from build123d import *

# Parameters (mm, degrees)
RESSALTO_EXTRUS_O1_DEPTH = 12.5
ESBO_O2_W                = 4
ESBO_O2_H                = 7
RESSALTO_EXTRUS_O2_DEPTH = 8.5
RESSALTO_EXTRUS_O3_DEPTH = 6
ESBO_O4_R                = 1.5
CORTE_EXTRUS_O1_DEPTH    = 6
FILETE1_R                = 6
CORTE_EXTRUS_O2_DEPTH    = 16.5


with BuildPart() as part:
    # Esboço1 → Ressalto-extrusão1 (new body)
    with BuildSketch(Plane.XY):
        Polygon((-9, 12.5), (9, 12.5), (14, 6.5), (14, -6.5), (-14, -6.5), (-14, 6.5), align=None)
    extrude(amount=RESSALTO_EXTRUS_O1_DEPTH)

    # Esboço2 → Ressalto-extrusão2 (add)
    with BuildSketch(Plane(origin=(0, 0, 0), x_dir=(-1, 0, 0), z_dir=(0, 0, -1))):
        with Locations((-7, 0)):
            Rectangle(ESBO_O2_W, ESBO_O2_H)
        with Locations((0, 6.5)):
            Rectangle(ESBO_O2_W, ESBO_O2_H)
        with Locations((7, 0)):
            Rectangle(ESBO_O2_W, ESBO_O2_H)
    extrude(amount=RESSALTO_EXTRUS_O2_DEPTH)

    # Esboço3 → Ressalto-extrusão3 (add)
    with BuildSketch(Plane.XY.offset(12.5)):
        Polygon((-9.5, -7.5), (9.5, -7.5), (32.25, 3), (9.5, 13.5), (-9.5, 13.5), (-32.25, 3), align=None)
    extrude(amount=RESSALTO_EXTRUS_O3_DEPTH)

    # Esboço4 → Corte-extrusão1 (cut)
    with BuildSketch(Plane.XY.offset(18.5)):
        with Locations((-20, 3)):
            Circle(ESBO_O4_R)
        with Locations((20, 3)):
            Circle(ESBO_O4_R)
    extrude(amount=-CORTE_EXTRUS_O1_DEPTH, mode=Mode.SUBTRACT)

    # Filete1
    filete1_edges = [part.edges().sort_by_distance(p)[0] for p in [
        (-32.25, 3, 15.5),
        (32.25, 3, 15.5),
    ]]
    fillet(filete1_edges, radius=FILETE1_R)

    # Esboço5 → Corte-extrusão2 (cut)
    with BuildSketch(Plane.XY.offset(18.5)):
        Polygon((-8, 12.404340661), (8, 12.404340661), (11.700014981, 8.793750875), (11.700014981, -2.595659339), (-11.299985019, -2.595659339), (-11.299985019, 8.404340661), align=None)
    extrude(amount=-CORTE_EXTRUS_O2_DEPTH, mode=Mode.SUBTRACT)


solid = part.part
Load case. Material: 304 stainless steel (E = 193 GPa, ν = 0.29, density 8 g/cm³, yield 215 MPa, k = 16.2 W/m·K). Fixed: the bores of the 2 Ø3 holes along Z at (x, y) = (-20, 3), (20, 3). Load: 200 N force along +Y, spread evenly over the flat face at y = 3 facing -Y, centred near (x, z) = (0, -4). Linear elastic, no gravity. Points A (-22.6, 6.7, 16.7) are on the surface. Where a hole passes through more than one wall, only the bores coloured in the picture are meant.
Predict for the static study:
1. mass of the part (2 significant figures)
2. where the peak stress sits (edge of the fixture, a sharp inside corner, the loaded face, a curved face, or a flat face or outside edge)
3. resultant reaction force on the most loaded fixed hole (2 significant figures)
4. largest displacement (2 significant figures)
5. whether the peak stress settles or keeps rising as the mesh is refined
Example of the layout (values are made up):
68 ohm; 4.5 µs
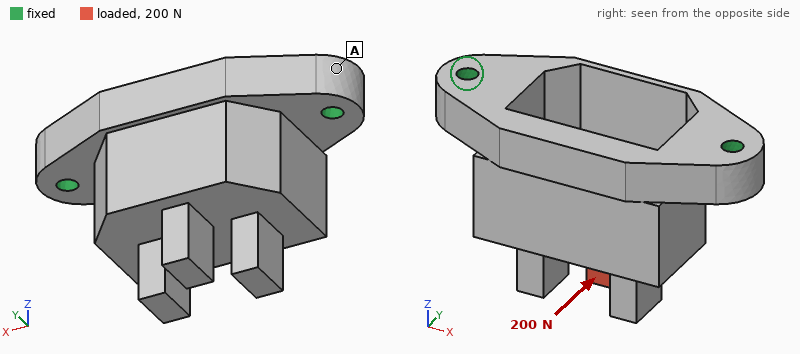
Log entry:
50 g; edge of the fixture; 110 N; 14 µm; keeps rising
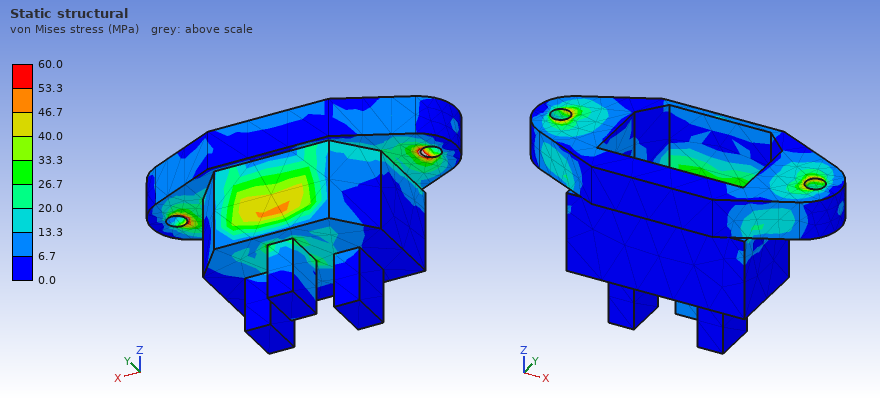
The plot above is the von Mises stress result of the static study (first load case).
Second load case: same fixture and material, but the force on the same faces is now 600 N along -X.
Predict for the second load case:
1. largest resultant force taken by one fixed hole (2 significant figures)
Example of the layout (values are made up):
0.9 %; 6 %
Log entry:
480 N
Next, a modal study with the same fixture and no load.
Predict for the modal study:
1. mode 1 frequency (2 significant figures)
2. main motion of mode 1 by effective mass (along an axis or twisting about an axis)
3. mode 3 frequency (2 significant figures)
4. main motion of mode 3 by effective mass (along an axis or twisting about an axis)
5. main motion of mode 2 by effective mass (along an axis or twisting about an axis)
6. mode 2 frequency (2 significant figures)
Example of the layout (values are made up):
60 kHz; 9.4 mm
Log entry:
6500 Hz; along Y; 14 kHz; along Z; along X; 13 kHz
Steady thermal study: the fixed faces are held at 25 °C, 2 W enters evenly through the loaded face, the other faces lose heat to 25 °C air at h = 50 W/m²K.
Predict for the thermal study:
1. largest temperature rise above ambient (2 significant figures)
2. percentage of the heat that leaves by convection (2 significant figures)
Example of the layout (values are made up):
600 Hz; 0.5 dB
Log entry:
45 K; 72 %
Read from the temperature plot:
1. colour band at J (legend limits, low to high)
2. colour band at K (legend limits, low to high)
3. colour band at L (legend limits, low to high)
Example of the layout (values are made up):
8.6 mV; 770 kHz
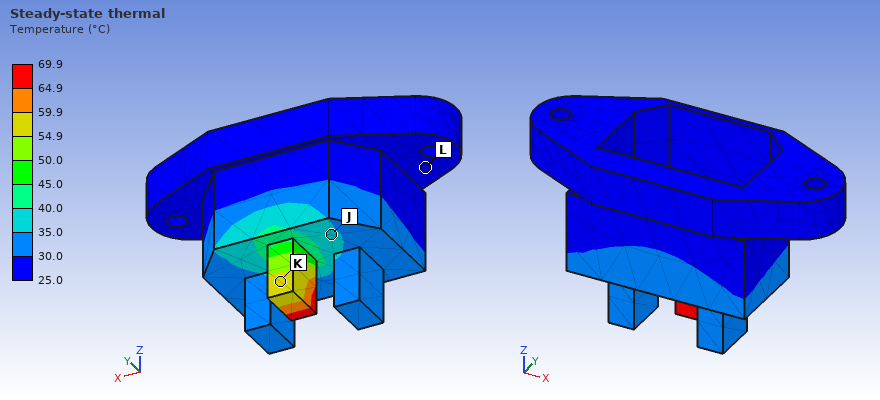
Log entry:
35.0 to 40.0 °C; 54.9 to 59.9 °C; 25.0 to 30.0 °C
